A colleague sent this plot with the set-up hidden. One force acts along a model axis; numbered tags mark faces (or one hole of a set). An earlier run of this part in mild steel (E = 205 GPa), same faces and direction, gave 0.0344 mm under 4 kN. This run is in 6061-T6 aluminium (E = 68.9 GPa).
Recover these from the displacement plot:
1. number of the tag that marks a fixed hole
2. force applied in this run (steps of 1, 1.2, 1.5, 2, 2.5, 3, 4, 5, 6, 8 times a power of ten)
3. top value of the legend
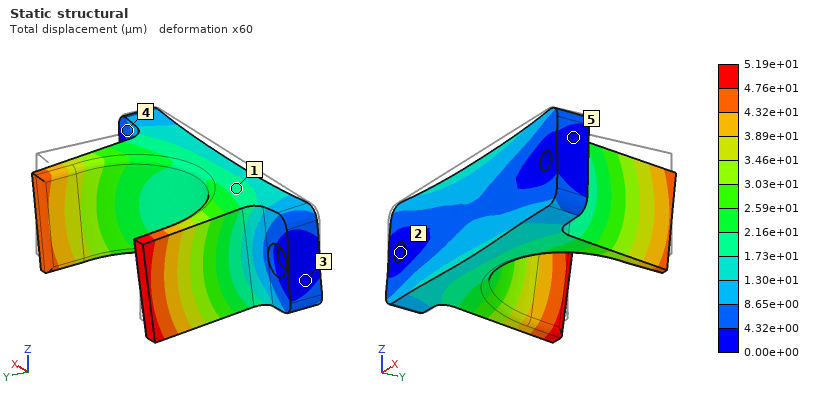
2
2 kN
5.19e+01 µm
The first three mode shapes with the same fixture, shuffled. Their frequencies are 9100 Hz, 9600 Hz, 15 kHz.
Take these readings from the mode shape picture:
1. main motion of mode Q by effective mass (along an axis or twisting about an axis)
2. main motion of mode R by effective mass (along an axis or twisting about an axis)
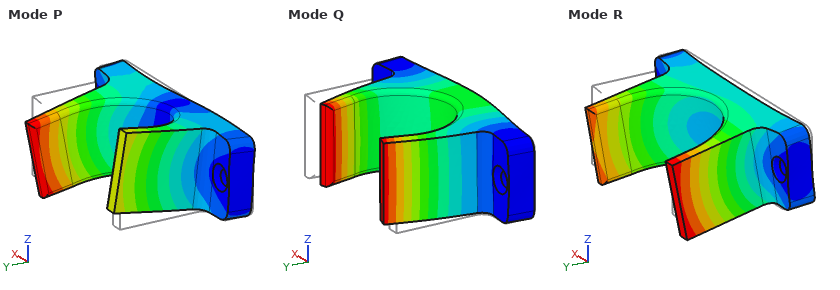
along Y
along Z
